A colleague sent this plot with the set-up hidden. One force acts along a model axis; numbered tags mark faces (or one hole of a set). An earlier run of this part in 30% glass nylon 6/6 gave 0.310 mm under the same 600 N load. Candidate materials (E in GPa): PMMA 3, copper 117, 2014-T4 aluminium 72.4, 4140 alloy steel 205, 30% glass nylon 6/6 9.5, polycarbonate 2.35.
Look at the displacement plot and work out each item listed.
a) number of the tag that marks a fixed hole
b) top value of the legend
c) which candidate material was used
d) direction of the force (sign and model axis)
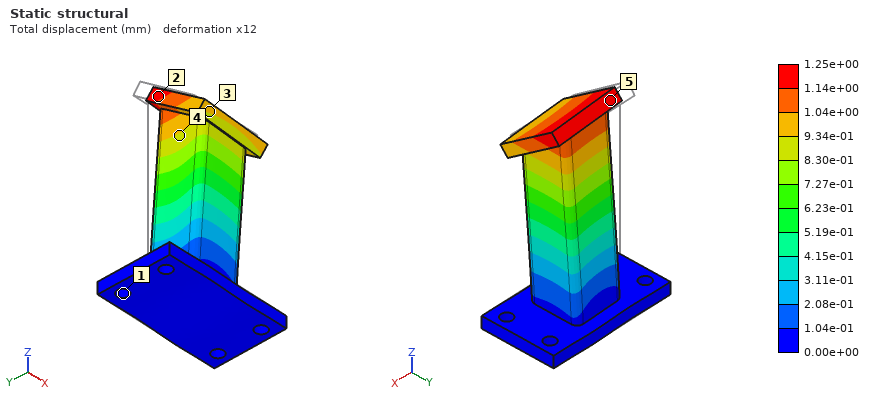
1
1.25e+00 mm
polycarbonate
+X
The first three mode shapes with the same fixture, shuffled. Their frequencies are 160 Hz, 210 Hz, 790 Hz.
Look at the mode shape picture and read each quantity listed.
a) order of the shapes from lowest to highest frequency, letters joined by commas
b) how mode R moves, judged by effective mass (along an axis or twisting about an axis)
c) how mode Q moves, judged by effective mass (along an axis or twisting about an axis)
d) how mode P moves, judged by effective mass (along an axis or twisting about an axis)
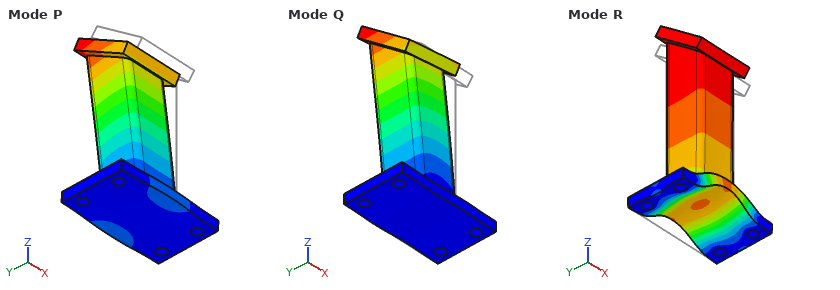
P, Q, R
along Z
along X
along Y
